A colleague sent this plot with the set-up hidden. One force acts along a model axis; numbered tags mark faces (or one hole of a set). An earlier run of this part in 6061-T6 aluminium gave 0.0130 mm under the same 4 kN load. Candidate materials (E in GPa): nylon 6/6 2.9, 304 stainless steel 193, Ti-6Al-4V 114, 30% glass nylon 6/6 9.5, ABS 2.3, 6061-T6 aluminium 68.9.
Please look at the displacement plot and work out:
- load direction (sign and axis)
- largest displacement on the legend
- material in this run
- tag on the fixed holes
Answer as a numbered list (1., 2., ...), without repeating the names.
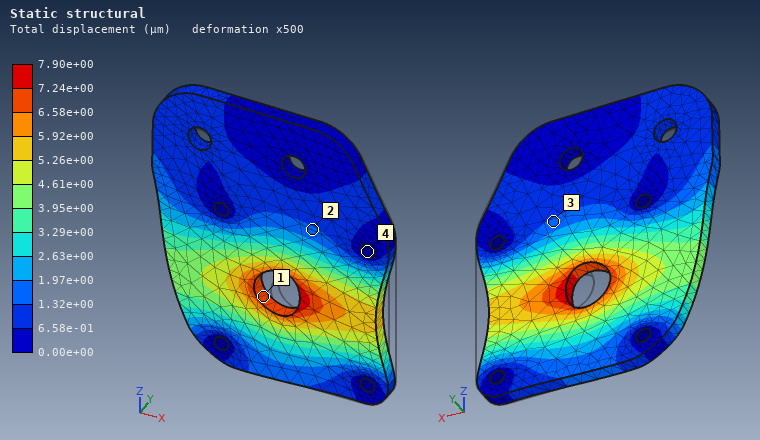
1. -X
2. 7.90e+00 µm
3. Ti-6Al-4V
4. 4
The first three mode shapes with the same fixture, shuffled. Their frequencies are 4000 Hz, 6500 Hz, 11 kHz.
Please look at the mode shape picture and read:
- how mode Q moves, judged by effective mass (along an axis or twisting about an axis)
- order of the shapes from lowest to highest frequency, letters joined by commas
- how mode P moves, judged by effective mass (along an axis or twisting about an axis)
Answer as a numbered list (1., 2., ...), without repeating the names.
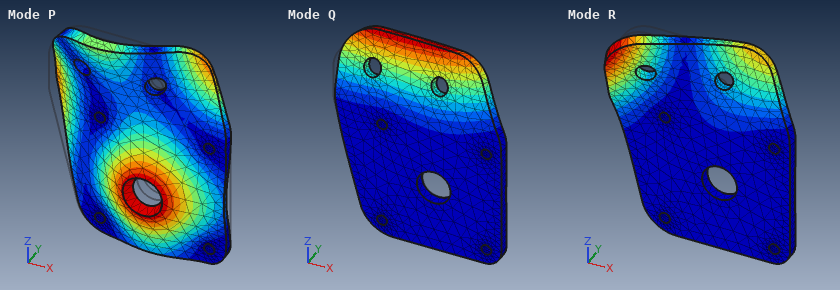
1. along Y
2. Q, R, P
3. along Y
